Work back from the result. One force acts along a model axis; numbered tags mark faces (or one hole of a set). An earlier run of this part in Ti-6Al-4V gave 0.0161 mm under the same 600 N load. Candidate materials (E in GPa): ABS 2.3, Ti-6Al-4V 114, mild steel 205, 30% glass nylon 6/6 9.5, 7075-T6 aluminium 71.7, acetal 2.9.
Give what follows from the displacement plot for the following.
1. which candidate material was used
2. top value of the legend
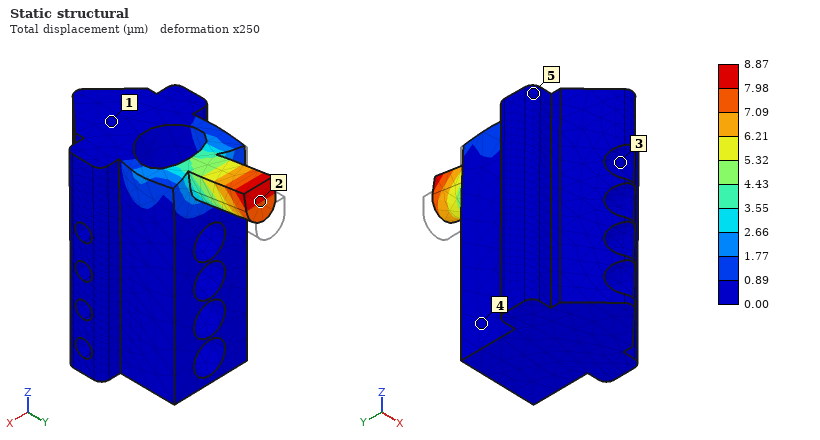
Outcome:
mild steel
8.87 µm
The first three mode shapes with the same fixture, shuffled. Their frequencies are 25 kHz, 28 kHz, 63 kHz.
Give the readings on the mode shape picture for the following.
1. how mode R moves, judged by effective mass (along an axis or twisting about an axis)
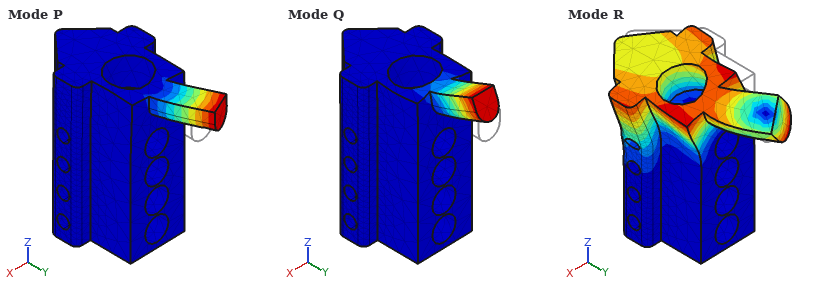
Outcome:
along X
